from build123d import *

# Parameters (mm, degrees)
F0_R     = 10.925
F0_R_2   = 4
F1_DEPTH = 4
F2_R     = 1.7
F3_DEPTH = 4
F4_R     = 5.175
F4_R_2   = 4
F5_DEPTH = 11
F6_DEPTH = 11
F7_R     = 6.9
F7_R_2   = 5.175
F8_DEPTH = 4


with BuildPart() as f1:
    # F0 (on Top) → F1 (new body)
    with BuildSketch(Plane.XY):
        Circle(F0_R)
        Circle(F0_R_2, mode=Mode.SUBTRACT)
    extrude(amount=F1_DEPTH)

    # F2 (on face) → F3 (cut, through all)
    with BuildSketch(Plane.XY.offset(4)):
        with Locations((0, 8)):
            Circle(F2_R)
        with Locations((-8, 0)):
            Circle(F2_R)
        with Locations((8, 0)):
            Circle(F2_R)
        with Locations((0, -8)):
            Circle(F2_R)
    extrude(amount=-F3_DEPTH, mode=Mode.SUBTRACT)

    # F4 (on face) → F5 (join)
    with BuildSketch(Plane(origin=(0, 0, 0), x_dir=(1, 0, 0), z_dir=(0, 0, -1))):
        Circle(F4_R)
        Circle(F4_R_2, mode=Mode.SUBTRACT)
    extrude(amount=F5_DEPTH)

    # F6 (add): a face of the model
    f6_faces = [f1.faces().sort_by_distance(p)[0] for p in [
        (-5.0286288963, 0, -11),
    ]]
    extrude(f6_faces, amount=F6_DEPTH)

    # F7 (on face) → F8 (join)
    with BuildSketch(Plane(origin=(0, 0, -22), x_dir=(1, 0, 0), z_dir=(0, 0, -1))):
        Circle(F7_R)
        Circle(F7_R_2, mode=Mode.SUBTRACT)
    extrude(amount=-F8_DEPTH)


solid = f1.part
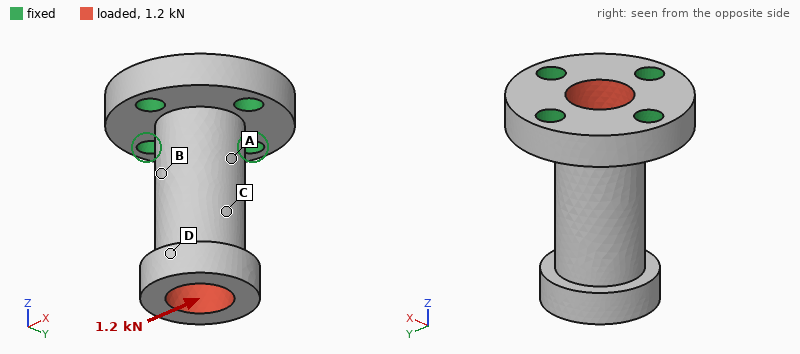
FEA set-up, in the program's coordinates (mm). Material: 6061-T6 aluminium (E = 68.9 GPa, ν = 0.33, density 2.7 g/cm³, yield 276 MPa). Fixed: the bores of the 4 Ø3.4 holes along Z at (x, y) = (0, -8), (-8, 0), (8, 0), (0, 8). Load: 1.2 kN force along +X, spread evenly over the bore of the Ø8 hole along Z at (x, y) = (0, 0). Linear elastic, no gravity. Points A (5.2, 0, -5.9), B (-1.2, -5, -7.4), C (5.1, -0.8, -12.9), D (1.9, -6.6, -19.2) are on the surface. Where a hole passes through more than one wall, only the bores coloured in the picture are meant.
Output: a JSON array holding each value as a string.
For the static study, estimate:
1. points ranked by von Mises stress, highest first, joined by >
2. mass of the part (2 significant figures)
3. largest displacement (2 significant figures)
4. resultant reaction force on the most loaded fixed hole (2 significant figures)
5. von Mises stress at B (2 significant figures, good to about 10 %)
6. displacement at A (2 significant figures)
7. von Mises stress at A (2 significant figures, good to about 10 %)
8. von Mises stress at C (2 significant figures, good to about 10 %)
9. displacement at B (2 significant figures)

["A > B > C > D", "5.8 g", "0.11 mm", "1.0 kN", "64 MPa", "0.032 mm", "82 MPa", "29 MPa", "0.032 mm"]
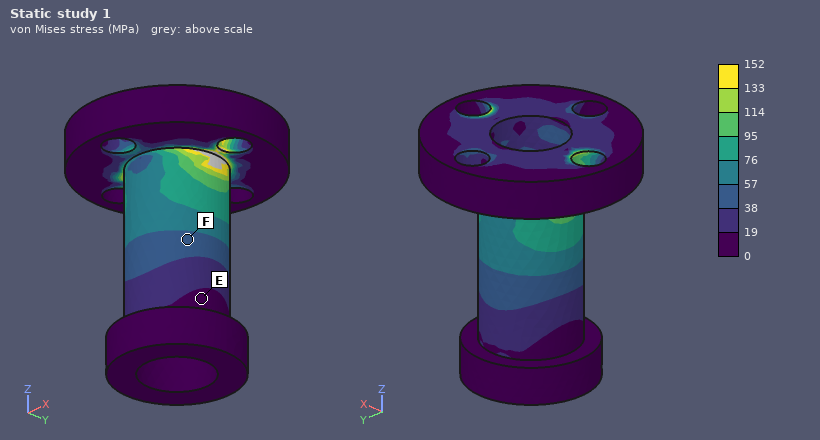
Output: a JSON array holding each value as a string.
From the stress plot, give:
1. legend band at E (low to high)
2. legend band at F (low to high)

["0 to 19 MPa", "38 to 57 MPa"]
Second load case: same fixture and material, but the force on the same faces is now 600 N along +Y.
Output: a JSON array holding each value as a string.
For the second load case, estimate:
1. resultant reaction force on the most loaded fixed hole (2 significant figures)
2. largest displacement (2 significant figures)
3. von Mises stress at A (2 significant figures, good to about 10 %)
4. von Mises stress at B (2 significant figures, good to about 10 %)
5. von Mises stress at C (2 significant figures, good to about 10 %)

["520 N", "54 µm", "35 MPa", "35 MPa", "19 MPa"]
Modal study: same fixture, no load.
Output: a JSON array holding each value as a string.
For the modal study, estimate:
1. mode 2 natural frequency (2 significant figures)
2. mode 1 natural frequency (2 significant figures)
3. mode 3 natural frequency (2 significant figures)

["9400 Hz", "9400 Hz", "23 kHz"]
